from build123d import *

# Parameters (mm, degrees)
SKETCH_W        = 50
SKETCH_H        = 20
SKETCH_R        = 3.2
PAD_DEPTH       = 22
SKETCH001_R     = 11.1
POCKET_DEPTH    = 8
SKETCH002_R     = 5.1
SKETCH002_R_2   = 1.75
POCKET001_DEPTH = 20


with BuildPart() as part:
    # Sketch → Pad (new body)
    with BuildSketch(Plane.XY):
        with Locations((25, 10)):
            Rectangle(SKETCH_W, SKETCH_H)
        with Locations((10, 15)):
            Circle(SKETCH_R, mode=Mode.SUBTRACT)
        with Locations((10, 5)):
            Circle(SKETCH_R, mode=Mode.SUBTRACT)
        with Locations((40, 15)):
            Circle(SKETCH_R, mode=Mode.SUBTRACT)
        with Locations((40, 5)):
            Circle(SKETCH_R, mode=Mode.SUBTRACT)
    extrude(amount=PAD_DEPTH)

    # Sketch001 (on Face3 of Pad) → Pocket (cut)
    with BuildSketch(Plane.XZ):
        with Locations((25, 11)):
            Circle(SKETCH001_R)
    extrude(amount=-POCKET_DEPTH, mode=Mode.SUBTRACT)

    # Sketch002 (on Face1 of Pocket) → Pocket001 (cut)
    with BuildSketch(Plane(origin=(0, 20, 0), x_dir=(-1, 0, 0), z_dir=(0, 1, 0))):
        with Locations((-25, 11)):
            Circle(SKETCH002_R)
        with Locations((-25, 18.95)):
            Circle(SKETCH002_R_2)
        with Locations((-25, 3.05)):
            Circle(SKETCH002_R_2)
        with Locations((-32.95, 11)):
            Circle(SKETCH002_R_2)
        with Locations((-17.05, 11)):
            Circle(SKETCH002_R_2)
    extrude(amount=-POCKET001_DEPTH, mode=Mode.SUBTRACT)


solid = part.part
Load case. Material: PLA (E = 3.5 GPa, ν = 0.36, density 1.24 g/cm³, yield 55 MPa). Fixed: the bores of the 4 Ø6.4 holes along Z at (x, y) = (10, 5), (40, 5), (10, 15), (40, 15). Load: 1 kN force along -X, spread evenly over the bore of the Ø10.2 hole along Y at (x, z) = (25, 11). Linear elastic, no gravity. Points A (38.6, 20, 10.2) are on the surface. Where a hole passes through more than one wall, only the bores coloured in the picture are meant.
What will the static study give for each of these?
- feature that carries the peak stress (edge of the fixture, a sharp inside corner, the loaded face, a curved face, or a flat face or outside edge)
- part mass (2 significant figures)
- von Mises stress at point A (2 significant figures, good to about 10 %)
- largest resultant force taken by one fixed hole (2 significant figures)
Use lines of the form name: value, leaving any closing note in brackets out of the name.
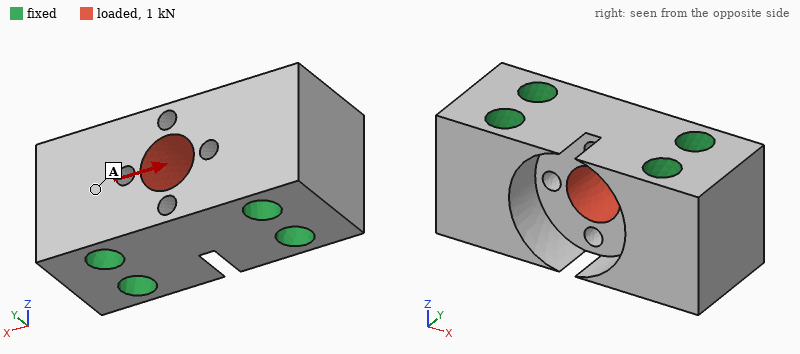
feature that carries the peak stress: a curved face
part mass: 18 g
von Mises stress at point A: 1.1 MPa
largest resultant force taken by one fixed hole: 400 N
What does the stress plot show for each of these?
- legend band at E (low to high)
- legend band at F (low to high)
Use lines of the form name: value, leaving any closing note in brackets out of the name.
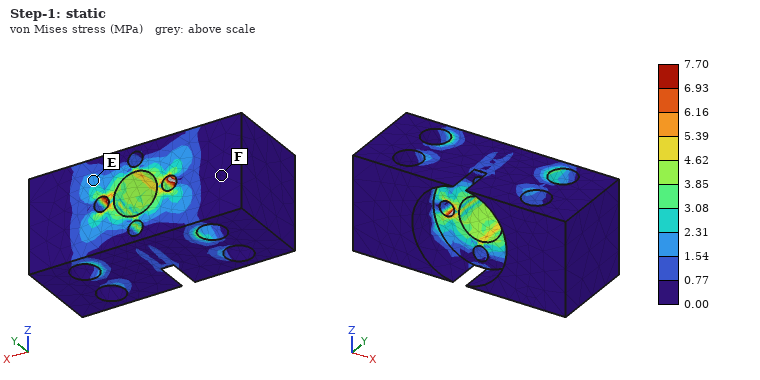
legend band at E: 1.54 to 2.31 MPa
legend band at F: 0.00 to 0.77 MPa
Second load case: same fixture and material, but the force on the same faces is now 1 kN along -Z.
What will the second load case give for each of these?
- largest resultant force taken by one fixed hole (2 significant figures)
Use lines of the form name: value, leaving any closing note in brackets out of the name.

largest resultant force taken by one fixed hole: 390 N
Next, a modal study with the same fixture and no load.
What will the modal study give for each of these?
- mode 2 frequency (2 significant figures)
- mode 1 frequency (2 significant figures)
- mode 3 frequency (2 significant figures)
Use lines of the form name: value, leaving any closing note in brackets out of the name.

mode 2 frequency: 20 kHz
mode 1 frequency: 20 kHz
mode 3 frequency: 22 kHz
